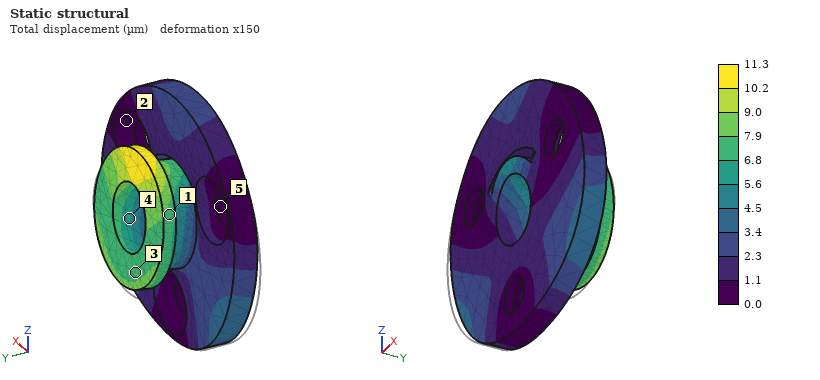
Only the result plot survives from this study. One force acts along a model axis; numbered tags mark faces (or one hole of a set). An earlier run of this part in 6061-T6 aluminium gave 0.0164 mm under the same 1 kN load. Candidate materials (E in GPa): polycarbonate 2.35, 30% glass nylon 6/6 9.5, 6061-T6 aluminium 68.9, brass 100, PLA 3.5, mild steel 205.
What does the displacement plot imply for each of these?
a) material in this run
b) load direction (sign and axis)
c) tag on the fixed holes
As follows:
brass
+Z
5
